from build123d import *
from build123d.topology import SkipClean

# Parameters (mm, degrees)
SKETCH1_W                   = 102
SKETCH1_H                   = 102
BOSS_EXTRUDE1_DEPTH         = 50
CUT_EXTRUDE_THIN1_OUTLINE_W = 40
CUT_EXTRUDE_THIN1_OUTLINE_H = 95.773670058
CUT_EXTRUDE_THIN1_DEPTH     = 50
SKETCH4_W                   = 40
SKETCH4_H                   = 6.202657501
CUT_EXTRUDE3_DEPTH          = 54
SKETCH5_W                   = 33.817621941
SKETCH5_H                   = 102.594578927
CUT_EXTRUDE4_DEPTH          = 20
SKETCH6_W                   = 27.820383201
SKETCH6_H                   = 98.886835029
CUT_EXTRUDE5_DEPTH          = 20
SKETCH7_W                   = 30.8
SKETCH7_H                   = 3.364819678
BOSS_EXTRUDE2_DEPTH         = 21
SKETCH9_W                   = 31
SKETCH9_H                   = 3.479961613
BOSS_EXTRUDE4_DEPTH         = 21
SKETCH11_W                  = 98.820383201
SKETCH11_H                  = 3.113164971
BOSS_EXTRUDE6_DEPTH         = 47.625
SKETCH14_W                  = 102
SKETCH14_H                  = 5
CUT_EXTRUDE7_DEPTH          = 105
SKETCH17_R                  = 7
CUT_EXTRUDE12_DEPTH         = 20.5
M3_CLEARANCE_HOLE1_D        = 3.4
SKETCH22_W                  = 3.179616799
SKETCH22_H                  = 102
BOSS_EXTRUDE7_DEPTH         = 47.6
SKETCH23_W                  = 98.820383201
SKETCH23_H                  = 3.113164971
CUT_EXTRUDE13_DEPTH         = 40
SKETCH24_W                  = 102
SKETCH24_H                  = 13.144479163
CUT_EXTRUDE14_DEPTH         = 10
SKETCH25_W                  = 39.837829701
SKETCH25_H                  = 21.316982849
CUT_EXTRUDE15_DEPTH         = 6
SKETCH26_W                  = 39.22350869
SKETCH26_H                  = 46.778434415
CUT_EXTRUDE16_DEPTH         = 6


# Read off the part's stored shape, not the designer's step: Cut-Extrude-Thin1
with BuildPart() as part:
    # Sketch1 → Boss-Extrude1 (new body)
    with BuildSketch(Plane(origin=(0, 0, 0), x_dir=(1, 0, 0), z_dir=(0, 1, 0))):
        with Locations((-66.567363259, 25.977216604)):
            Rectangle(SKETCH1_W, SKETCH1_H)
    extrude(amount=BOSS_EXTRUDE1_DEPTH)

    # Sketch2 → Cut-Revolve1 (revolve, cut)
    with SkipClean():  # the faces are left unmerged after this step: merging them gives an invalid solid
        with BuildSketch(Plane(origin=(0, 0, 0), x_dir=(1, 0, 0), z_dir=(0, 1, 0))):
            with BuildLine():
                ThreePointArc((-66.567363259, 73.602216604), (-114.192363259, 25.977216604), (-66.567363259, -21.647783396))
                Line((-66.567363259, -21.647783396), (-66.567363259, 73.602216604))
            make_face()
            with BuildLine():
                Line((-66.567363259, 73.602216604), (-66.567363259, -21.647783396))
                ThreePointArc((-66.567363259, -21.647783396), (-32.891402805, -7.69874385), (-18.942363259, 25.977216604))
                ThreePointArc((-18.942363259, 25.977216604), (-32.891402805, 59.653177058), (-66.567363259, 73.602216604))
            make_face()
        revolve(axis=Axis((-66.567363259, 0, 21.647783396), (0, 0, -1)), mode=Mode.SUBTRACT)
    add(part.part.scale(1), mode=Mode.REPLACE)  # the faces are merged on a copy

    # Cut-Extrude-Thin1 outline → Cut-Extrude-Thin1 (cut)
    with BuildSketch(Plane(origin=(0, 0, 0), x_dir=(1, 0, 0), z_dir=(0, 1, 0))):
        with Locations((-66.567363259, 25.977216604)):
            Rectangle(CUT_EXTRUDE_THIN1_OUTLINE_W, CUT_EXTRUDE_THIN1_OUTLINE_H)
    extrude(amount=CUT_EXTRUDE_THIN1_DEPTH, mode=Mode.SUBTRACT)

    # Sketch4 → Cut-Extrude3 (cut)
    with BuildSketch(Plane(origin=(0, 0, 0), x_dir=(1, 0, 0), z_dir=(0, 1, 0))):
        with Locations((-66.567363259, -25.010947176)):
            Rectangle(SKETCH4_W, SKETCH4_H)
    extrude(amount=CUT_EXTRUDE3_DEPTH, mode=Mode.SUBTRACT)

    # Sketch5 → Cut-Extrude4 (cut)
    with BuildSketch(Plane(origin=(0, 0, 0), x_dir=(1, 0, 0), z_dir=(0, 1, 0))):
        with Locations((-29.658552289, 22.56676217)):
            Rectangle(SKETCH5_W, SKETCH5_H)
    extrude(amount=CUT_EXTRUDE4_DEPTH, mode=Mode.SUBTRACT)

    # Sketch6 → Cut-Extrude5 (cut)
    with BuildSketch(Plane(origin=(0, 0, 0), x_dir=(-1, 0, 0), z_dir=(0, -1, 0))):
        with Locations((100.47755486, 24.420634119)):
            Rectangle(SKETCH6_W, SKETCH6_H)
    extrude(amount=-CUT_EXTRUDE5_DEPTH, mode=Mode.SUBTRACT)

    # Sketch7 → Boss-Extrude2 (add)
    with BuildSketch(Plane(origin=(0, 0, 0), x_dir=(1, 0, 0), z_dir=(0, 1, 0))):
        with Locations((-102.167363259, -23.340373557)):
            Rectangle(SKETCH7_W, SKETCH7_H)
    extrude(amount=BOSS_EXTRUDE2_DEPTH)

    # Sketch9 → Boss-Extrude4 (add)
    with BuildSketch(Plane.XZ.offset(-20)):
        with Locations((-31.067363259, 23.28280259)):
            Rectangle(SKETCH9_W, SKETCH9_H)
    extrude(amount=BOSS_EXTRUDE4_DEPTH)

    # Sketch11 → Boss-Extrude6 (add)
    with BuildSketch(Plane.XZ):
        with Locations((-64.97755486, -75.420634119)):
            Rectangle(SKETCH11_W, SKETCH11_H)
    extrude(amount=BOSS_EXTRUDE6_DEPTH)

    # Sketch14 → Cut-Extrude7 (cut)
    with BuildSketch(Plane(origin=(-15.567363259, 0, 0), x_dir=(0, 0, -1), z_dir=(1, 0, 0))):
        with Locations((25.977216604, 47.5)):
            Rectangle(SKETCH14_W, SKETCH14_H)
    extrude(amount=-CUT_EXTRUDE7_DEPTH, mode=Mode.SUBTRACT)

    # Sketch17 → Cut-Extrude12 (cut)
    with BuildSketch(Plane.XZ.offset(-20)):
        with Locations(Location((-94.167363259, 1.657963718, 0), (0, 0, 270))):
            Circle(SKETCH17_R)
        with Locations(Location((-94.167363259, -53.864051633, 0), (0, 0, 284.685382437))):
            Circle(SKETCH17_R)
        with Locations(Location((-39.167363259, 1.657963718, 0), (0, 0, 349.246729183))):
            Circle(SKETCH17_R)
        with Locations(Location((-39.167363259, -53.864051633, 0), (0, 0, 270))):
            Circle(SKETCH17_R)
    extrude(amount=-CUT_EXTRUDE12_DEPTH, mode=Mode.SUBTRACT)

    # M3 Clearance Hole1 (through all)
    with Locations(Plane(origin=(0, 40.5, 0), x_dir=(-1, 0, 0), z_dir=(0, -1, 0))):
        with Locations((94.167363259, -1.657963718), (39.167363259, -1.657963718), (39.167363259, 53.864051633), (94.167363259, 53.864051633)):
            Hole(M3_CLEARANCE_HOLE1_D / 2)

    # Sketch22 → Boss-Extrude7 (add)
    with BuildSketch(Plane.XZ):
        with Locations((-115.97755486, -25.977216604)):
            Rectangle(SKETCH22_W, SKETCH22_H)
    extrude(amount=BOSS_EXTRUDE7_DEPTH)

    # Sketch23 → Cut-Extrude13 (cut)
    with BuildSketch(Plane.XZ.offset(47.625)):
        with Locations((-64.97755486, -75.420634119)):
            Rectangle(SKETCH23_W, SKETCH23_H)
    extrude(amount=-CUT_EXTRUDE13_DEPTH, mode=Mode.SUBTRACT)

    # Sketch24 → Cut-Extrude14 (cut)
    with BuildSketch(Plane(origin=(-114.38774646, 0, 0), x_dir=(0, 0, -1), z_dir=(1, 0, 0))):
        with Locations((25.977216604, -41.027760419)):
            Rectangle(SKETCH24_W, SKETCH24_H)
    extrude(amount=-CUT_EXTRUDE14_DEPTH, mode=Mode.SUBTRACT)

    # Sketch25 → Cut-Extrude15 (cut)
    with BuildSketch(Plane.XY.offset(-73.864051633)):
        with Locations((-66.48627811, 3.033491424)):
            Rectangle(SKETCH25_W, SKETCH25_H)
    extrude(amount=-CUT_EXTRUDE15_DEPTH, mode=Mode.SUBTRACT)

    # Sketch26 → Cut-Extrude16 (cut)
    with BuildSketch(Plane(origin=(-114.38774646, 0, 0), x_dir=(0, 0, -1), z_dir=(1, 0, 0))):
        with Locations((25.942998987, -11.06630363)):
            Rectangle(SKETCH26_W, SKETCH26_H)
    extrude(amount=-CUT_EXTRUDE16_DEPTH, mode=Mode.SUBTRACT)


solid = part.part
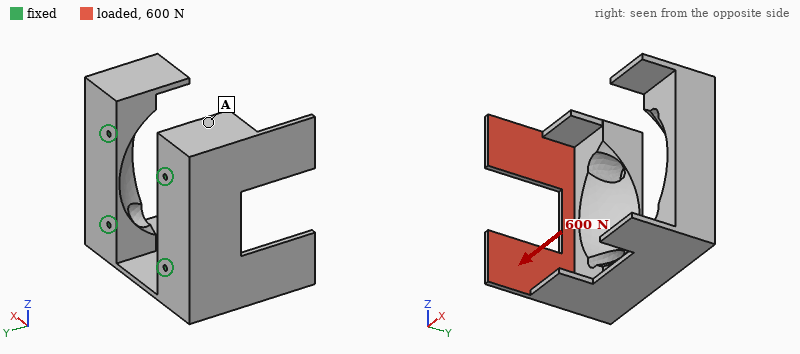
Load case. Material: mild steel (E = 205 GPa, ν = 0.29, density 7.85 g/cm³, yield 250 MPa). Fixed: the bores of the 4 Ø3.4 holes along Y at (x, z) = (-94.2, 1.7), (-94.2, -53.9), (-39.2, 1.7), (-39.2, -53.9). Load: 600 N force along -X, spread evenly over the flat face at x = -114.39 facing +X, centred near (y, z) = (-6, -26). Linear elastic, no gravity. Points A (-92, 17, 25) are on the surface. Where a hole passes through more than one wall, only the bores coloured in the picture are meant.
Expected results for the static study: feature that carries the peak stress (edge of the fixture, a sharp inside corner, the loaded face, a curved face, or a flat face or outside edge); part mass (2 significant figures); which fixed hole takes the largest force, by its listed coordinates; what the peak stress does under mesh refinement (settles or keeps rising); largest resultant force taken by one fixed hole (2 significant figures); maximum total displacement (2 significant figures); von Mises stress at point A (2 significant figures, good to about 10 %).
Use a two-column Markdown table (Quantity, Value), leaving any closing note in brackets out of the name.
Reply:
| Quantity | Value |
|---|---|
| feature that carries the peak stress | edge of the fixture |
| part mass | 1.1 kg |
| which fixed hole takes the largest force, by its listed coordinates | (-39.2, -53.9) |
| what the peak stress does under mesh refinement | keeps rising |
| largest resultant force taken by one fixed hole | 610 N |
| maximum total displacement | 0.22 mm |
| von Mises stress at point A | 13 MPa |
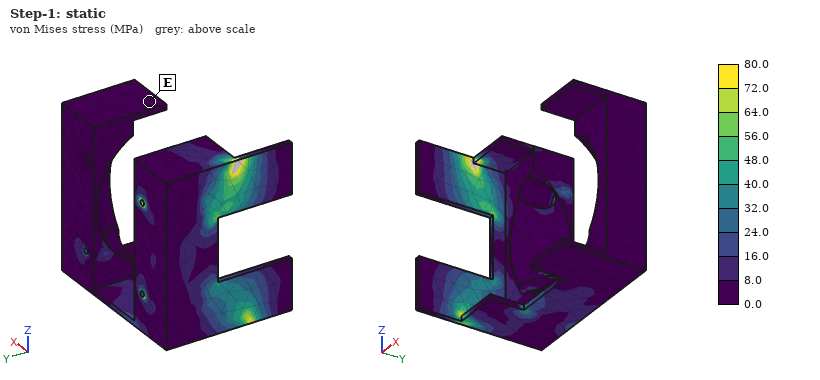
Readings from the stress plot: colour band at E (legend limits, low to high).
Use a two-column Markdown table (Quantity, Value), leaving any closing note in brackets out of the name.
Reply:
| Quantity | Value |
|---|---|
| colour band at E | 0.0 to 8.0 MPa |
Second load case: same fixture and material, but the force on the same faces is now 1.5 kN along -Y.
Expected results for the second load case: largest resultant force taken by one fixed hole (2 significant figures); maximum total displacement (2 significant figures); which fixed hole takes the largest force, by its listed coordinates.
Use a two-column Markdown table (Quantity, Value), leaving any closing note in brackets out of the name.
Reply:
| Quantity | Value |
|---|---|
| largest resultant force taken by one fixed hole | 1.3 kN |
| maximum total displacement | 34 µm |
| which fixed hole takes the largest force, by its listed coordinates | (-94.2, -53.9) |
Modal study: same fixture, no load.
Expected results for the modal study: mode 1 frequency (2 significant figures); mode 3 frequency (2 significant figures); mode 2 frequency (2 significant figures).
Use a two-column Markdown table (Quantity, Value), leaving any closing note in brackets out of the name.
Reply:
| Quantity | Value |
|---|---|
| mode 1 frequency | 1200 Hz |
| mode 3 frequency | 2400 Hz |
| mode 2 frequency | 1500 Hz |
